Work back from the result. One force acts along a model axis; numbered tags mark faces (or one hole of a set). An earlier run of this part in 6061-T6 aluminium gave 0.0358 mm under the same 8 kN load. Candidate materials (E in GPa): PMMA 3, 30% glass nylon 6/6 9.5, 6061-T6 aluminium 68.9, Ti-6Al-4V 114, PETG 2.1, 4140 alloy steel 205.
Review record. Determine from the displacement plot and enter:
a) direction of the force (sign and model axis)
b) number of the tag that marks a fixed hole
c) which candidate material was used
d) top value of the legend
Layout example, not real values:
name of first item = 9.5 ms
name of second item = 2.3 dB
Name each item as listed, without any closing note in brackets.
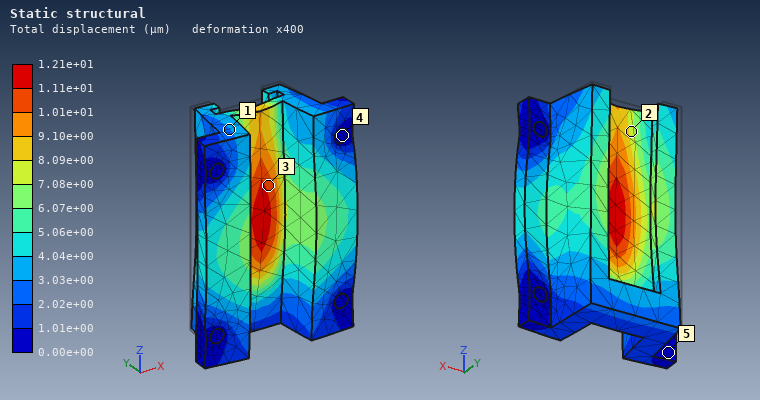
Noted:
direction of the force = -Y
number of the tag that marks a fixed hole = 4
which candidate material was used = 4140 alloy steel
top value of the legend = 1.21e+01 µm
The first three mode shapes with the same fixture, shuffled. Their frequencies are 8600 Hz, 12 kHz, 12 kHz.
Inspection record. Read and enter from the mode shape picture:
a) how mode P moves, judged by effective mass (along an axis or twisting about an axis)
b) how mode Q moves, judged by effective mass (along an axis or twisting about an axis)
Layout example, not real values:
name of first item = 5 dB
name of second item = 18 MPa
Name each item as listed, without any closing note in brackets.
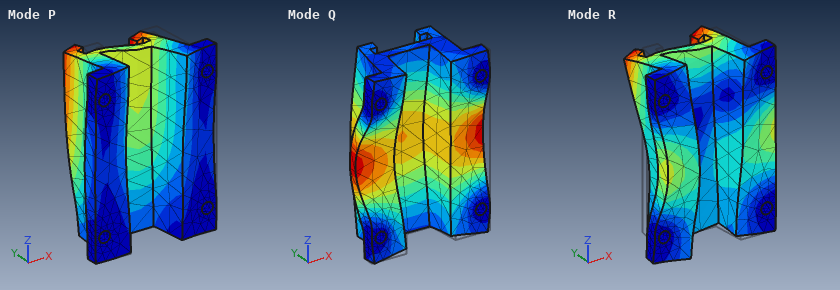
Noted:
how mode P moves, judged by effective mass = along X
how mode Q moves, judged by effective mass = along Y
